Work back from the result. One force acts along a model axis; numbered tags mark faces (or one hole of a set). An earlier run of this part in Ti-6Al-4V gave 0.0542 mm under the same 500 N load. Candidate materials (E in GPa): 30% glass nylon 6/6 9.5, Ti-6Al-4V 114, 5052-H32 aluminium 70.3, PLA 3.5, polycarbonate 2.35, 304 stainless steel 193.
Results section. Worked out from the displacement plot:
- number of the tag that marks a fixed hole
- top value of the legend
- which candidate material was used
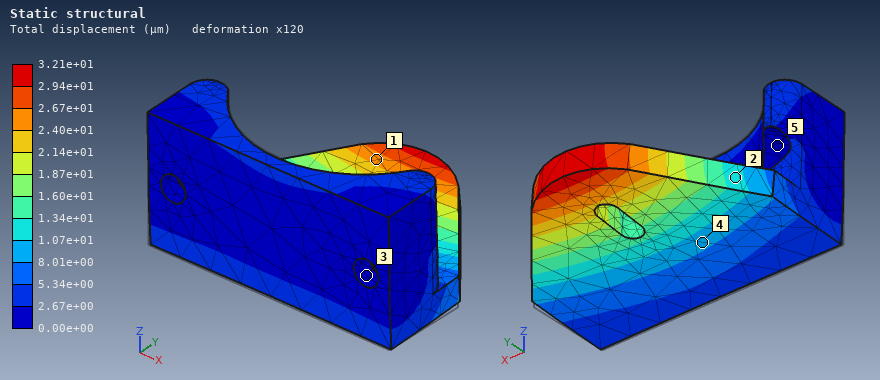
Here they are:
3
3.21e+01 µm
304 stainless steel
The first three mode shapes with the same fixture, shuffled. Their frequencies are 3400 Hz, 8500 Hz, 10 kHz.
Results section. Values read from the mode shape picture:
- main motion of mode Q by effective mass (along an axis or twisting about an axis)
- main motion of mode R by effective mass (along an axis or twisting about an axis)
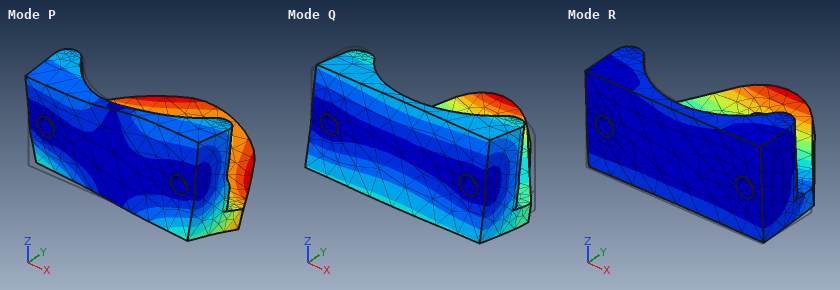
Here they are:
along Y
along Z
